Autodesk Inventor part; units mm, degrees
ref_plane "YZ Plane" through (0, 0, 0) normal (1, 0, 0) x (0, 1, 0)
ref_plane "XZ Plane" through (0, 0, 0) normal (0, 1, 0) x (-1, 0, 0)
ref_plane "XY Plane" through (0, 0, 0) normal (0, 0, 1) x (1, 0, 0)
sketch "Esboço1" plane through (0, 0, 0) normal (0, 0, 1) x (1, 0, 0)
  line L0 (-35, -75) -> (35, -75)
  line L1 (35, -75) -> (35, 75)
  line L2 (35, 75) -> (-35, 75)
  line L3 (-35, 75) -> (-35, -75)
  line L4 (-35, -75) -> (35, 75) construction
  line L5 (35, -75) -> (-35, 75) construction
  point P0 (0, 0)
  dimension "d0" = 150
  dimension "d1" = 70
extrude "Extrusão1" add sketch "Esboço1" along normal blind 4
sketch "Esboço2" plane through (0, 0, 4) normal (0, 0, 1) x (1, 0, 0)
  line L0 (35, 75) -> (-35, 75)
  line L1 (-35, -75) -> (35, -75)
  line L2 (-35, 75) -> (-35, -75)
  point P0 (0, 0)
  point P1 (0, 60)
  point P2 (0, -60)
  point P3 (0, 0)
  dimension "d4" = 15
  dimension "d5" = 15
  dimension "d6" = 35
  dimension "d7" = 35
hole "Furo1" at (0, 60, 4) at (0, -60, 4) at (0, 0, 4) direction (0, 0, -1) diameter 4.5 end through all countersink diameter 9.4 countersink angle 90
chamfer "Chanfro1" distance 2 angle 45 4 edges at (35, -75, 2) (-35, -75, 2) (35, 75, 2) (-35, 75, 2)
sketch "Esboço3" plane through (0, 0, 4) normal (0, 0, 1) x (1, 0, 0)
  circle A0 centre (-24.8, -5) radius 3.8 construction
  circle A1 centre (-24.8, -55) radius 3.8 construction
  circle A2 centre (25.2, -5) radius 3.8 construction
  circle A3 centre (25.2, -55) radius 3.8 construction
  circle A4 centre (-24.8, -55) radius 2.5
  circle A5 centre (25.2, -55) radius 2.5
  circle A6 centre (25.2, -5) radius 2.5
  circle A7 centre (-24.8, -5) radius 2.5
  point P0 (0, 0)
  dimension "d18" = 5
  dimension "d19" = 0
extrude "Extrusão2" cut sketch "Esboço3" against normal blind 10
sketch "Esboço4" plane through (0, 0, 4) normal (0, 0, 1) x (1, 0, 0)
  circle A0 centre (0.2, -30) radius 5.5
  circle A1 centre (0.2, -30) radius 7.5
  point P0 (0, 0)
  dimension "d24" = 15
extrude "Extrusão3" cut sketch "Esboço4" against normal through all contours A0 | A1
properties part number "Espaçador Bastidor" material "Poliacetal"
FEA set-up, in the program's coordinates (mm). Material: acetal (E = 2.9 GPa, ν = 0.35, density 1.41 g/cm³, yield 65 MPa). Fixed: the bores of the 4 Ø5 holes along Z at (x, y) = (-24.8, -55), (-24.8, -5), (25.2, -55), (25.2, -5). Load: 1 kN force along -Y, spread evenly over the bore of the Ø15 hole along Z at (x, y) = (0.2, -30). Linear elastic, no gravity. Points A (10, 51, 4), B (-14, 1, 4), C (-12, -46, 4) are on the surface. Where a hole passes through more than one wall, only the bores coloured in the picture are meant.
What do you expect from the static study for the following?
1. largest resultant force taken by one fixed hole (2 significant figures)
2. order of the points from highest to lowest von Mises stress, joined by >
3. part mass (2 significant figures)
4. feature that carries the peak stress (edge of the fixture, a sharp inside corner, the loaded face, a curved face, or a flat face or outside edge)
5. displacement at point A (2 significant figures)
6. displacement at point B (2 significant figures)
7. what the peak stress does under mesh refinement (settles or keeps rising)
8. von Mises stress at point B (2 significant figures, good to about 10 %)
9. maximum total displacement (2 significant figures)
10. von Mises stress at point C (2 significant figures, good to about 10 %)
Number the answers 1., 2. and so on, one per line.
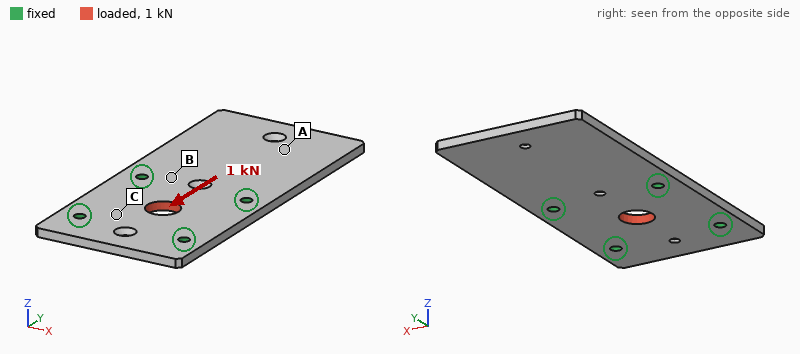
1. 270 N
2. C > B > A
3. 57 g
4. edge of the fixture
5. 13 µm
6. 15 µm
7. keeps rising
8. 1.7 MPa
9. 51 µm
10. 3.5 MPa
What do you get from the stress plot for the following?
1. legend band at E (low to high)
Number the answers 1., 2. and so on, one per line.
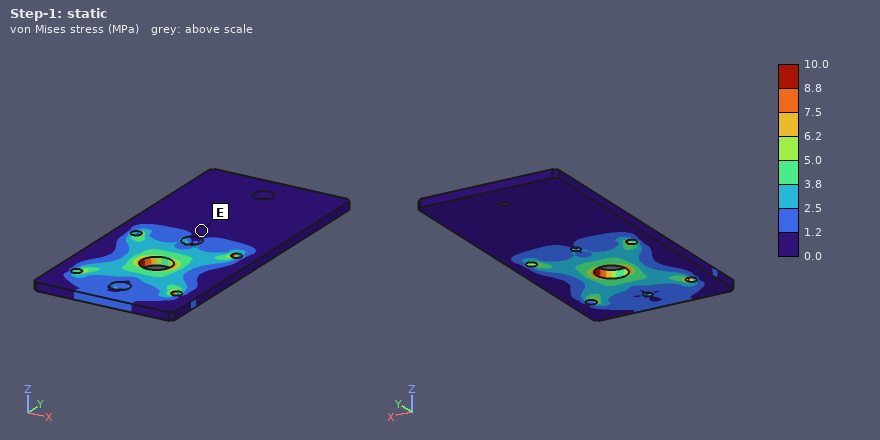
1. 0.0 to 1.2 MPa
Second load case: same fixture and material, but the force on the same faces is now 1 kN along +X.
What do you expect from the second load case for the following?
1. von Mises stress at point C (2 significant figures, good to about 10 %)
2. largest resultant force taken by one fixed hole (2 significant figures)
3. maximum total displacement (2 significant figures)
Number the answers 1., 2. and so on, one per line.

1. 3.9 MPa
2. 280 N
3. 57 µm
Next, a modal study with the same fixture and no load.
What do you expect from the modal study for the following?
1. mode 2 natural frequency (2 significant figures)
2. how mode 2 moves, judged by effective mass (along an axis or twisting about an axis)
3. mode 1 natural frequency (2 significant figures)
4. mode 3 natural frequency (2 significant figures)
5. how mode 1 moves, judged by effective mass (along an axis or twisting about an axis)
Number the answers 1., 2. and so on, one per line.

1. 390 Hz
2. twisting about Y
3. 140 Hz
4. 880 Hz
5. along Z
